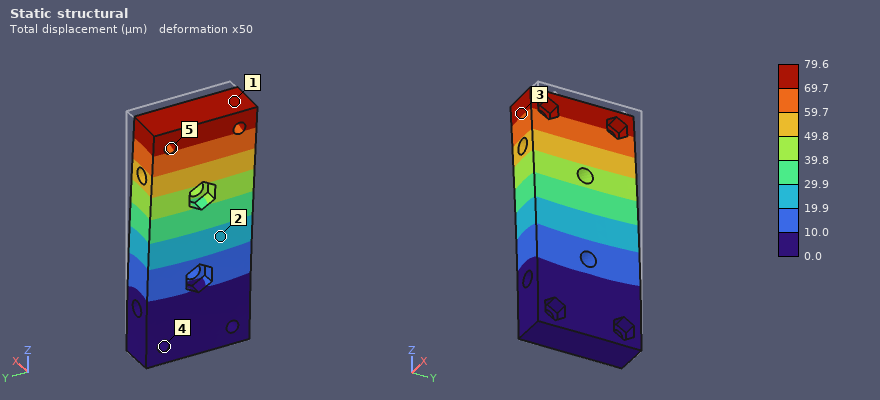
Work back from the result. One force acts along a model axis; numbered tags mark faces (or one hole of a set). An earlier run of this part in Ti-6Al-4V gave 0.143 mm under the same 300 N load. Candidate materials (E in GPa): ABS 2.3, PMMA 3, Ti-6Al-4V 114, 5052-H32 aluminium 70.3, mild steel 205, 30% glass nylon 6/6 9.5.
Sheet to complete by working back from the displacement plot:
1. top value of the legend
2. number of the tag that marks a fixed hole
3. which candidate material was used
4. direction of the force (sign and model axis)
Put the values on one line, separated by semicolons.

79.6 µm; 4; mild steel; -X
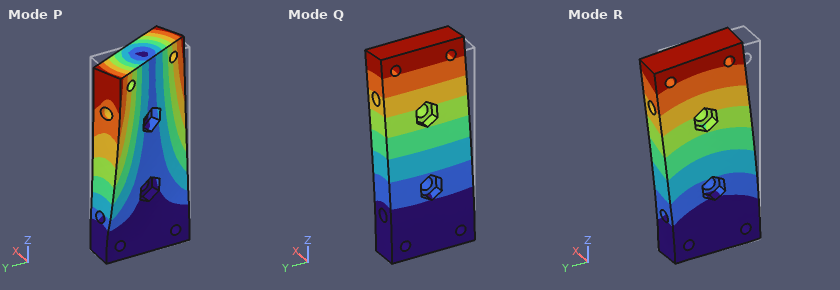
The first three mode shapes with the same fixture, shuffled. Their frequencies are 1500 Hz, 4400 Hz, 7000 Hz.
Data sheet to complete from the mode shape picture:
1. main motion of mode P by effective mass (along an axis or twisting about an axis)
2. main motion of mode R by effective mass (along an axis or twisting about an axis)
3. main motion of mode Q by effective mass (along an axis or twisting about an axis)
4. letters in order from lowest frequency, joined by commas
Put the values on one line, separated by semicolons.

twisting about Z; along Y; along X; Q, R, P
